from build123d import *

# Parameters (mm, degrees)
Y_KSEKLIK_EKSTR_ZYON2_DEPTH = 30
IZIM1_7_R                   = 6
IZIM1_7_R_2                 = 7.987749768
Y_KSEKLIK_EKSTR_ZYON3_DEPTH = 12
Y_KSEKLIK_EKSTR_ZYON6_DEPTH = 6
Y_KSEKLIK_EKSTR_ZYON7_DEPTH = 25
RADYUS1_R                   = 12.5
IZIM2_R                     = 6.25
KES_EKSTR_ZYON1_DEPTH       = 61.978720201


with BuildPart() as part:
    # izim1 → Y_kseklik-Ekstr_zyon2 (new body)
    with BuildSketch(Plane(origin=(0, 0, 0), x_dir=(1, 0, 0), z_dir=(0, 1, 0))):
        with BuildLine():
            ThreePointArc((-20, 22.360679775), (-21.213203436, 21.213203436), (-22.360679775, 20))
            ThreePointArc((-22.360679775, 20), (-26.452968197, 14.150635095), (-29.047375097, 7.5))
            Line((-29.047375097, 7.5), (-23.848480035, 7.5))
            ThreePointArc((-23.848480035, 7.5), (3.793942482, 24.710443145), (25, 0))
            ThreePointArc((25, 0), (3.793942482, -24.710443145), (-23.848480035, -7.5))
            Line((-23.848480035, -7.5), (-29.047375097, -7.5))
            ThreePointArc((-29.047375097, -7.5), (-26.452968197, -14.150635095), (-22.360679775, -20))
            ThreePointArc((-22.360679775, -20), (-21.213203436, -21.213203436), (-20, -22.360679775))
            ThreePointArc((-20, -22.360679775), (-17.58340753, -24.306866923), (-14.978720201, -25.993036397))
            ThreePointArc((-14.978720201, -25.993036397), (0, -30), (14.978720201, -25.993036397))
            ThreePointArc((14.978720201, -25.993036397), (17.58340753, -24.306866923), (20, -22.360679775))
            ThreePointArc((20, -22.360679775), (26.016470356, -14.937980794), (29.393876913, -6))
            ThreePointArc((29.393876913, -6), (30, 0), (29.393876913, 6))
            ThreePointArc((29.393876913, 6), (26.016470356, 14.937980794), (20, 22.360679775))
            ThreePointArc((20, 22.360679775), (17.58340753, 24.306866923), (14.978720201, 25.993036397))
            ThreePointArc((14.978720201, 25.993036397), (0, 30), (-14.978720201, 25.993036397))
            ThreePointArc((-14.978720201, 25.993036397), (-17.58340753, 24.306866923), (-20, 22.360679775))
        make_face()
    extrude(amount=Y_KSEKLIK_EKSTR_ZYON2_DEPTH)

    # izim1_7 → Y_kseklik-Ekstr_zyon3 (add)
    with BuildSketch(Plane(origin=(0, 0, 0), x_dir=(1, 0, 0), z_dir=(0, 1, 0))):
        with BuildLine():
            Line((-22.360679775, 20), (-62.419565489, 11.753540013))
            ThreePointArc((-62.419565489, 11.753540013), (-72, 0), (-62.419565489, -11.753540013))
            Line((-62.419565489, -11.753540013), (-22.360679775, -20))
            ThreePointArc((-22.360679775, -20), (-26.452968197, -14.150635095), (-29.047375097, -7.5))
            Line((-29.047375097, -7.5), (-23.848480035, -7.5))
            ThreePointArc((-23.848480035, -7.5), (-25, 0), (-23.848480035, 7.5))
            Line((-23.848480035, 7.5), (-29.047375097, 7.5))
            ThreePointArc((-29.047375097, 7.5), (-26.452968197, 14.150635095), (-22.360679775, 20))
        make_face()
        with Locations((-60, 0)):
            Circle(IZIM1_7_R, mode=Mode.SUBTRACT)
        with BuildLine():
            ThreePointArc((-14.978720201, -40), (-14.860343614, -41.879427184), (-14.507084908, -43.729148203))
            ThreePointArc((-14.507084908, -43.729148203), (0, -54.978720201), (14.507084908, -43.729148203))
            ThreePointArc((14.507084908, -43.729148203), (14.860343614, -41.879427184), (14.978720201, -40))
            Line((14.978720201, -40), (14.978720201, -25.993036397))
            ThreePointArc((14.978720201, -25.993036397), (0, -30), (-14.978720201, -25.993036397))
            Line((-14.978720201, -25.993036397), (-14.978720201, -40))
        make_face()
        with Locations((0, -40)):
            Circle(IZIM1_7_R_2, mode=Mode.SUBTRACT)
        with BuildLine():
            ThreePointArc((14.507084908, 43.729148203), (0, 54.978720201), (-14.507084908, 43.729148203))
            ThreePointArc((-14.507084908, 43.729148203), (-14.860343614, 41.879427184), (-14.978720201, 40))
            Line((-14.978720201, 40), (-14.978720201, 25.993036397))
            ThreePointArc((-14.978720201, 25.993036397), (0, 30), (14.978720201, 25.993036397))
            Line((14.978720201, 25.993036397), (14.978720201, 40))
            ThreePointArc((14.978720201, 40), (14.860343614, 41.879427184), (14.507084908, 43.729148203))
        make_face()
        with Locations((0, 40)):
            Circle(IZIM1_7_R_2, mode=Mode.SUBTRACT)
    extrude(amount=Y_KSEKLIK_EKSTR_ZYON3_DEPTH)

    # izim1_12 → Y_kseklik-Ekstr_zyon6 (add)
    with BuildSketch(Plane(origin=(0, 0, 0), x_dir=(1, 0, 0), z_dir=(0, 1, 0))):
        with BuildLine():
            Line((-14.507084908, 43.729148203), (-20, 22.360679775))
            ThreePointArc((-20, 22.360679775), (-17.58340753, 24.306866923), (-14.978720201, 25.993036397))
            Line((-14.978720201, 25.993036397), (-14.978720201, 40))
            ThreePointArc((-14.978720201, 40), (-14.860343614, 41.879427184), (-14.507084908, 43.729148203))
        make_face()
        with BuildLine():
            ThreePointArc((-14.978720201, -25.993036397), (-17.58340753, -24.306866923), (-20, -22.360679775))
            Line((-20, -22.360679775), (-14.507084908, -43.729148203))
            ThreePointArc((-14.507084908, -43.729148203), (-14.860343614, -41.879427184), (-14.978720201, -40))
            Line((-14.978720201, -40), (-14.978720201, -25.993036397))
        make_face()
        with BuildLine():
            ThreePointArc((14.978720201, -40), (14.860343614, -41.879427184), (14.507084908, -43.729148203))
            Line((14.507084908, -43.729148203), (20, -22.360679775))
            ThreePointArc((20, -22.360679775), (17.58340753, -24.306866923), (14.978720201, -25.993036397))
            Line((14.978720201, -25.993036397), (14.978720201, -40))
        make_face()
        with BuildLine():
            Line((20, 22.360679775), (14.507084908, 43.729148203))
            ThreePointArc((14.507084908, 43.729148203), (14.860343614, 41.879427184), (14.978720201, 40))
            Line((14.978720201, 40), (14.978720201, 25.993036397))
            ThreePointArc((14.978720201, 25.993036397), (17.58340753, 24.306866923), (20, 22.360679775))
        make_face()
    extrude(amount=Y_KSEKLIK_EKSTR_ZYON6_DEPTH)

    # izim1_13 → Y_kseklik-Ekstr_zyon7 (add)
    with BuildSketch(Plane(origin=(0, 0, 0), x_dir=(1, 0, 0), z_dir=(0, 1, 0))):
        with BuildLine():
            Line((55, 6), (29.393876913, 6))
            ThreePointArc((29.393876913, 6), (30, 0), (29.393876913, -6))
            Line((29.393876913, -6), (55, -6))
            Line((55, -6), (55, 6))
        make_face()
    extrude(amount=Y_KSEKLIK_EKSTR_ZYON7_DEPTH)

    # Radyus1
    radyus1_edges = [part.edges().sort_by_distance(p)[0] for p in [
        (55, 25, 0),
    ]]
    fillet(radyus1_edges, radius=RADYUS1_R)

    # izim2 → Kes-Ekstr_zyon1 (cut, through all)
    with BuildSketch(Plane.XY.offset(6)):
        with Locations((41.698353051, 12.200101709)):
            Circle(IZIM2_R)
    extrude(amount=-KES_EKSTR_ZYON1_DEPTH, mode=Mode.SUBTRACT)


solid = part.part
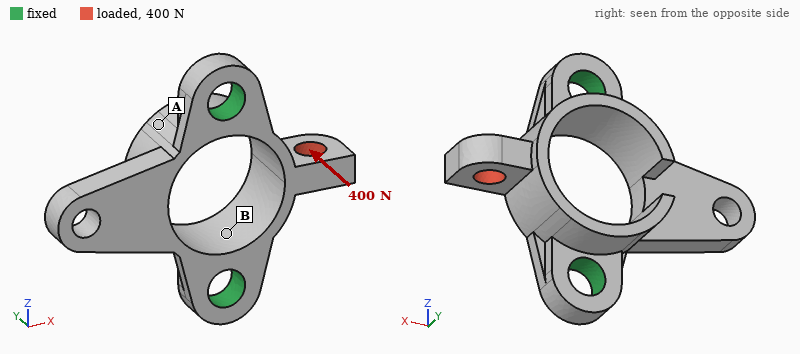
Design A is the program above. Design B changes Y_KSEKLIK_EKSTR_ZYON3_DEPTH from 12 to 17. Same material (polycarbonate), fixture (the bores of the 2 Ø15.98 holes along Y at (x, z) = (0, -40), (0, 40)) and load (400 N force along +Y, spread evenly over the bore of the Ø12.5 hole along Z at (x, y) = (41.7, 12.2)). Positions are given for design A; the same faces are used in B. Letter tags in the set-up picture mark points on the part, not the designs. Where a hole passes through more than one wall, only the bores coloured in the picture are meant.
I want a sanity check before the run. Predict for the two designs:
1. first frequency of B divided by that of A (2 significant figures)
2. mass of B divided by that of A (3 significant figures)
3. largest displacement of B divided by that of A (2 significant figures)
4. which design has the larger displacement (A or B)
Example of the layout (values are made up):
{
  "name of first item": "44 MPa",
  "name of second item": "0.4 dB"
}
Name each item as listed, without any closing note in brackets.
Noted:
{
  "first frequency of B divided by that of A": "1.2",
  "mass of B divided by that of A": "1.19",
  "largest displacement of B divided by that of A": "0.75",
  "which design has the larger displacement": "A"
}
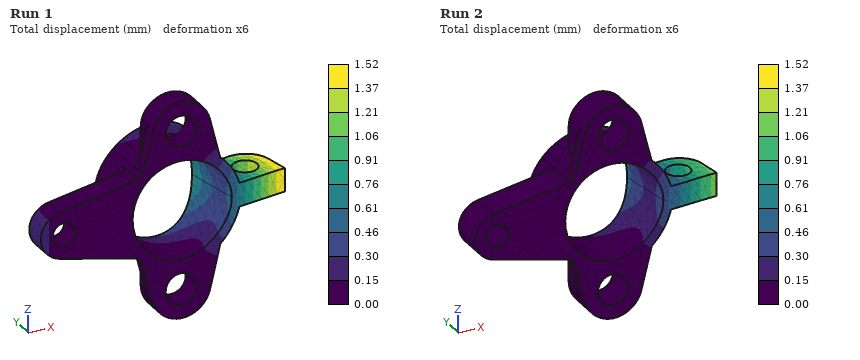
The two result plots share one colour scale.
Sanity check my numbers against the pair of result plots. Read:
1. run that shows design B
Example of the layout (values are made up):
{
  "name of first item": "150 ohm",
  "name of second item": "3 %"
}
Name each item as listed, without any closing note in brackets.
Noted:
{
  "run that shows design B": "Run 2"
}
